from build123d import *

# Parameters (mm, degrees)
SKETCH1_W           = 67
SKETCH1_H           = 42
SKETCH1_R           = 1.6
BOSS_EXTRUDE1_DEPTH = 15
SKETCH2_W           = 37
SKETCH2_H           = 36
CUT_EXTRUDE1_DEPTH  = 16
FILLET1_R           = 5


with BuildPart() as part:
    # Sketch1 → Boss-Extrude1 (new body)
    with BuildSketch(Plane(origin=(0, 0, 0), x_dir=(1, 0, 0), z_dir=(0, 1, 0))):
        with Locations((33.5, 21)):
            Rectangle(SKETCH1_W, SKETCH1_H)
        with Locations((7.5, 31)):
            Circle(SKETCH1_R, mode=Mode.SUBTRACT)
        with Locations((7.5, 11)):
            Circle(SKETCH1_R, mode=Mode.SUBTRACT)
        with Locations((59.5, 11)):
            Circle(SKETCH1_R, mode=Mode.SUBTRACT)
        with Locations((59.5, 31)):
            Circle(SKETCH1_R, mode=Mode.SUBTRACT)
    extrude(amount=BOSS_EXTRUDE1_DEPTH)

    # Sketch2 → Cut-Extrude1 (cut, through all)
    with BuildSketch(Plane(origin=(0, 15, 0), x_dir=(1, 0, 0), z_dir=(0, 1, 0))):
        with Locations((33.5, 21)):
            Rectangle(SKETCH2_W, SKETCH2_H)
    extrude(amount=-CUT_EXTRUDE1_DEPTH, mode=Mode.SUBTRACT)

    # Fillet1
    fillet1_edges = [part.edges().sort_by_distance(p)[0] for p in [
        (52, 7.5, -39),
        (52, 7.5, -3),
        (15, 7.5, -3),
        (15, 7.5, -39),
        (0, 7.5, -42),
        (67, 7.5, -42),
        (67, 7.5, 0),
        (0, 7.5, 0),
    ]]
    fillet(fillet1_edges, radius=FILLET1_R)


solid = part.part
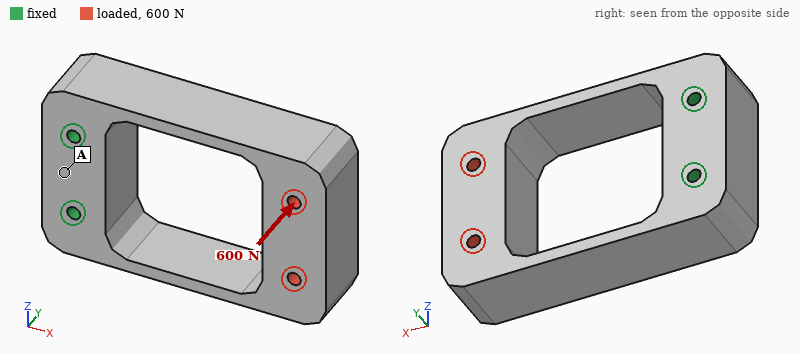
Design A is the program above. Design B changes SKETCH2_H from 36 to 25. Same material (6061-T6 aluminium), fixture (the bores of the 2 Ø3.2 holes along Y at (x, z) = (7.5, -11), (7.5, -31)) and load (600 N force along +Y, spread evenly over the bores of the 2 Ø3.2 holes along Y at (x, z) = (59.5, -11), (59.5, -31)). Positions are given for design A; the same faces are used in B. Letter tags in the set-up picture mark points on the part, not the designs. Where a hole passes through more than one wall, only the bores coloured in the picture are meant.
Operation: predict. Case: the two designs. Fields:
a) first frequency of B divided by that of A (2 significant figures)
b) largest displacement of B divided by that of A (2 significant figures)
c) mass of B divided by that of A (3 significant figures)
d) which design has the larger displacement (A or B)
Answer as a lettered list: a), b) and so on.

a) 2.1
b) 0.41
c) 1.28
d) A
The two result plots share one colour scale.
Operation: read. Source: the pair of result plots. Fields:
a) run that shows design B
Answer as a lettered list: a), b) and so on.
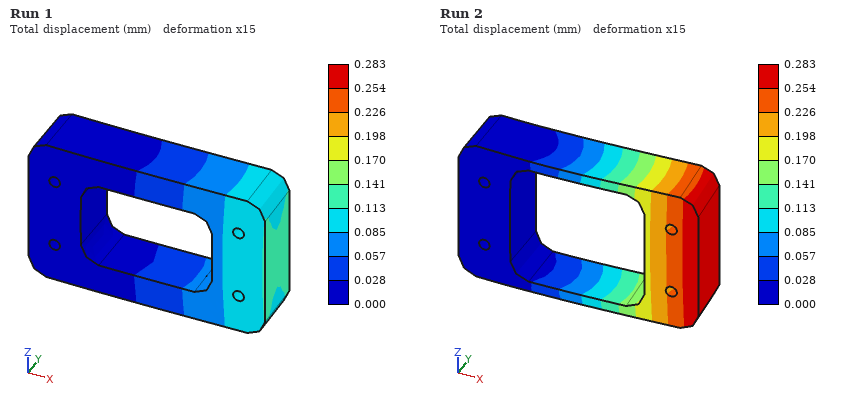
a) Run 1
